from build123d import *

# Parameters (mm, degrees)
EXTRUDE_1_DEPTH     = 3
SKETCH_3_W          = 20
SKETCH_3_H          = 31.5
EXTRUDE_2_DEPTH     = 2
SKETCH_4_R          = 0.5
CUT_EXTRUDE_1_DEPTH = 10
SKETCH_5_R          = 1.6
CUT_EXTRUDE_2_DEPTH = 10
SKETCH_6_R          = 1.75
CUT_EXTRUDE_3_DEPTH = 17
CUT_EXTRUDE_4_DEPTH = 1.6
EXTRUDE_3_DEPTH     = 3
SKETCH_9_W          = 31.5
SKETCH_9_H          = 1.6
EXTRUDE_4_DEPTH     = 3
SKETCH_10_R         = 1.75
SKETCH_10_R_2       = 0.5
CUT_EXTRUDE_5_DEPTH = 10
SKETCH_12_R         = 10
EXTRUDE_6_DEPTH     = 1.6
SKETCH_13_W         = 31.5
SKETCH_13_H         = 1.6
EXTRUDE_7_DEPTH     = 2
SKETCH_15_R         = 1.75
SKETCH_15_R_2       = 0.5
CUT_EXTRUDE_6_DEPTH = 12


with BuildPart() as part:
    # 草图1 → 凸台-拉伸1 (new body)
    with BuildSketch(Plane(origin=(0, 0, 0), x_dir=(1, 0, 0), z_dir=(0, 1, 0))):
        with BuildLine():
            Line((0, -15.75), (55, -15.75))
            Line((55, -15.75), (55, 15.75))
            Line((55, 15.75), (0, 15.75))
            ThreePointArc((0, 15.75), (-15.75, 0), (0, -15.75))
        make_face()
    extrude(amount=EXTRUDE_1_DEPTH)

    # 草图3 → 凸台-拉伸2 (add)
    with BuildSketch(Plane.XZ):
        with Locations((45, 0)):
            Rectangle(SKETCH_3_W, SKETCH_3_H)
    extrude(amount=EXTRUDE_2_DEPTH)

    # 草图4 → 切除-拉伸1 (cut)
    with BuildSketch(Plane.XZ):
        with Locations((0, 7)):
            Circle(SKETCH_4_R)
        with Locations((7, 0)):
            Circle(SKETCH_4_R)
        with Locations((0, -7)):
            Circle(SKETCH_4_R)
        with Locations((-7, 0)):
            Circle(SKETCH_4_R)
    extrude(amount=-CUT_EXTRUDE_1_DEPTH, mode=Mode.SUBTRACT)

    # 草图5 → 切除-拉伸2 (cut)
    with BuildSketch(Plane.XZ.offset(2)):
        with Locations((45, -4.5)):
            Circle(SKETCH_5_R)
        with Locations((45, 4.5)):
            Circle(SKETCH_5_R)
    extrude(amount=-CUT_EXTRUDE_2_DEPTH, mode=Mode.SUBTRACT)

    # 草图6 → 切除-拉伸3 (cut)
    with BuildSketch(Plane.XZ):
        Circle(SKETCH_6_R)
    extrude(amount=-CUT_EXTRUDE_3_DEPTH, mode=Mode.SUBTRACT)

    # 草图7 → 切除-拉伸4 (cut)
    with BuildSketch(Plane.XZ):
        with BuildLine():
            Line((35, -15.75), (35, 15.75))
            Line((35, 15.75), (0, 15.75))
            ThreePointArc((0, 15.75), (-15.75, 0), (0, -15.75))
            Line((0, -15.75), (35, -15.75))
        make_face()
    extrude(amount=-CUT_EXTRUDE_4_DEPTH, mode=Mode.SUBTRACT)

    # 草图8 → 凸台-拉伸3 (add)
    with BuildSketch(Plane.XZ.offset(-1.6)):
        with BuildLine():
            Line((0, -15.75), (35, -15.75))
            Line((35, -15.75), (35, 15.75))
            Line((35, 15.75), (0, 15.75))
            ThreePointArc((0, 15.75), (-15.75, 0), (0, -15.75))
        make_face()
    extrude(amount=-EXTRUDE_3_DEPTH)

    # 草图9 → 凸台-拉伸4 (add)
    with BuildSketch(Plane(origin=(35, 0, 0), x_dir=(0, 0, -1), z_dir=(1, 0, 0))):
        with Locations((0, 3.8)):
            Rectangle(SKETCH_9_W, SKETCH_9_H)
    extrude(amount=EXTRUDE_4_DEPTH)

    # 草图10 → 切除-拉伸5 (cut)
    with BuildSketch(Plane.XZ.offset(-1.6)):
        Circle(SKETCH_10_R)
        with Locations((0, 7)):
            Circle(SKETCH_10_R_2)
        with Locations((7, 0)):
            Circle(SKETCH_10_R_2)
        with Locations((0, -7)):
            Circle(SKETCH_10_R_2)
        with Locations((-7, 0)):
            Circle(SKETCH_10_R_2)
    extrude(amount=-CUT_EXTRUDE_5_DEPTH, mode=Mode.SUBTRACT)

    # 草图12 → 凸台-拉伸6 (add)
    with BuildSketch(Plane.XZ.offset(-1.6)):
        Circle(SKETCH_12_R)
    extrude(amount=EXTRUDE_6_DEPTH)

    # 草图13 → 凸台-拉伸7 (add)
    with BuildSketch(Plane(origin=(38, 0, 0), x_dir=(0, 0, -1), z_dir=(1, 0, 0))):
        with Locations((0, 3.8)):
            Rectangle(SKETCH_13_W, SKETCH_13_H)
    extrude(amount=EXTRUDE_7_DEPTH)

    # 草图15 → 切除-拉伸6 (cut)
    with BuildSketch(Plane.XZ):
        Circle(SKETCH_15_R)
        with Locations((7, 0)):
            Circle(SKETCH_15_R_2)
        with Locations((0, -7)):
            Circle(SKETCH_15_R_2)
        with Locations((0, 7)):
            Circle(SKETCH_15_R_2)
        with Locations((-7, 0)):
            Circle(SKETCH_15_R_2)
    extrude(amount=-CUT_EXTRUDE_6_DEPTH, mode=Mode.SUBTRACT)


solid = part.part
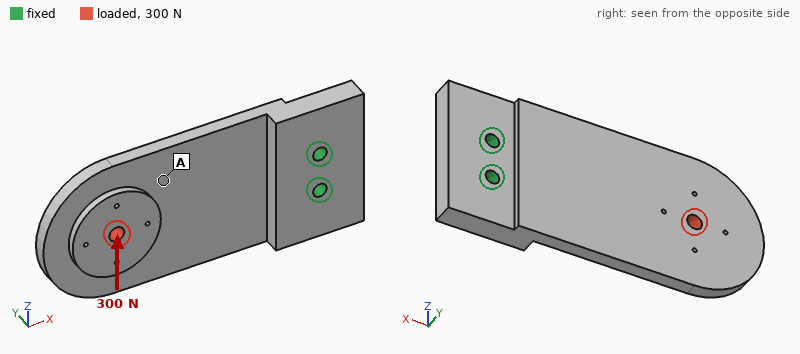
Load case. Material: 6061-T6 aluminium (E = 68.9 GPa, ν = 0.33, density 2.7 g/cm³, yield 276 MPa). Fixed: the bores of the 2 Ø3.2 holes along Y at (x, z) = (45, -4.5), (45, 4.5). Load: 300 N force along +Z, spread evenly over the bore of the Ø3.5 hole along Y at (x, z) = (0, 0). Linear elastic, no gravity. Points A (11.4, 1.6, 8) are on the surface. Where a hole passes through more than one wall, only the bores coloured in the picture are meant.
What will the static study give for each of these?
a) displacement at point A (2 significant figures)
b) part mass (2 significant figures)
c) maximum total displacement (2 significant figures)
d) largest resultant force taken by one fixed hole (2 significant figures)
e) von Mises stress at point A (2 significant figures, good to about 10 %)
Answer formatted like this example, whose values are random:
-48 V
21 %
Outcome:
32 µm
22 g
56 µm
1.2 kN
11 MPa
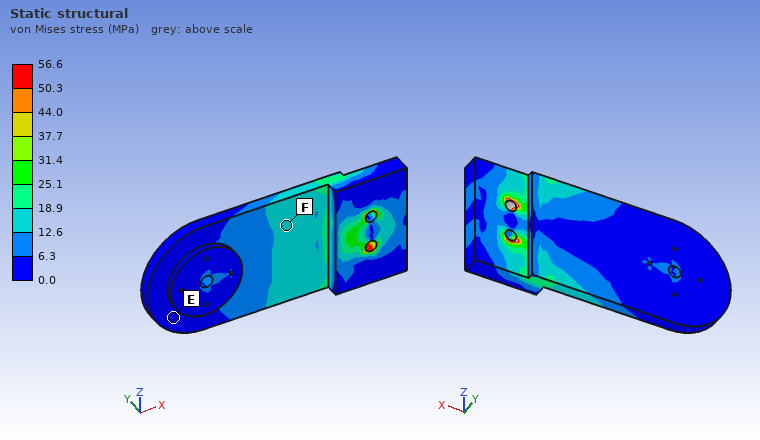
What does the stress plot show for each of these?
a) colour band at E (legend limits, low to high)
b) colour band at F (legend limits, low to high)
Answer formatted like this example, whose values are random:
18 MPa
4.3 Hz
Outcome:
0.0 to 6.3 MPa
12.6 to 18.9 MPa
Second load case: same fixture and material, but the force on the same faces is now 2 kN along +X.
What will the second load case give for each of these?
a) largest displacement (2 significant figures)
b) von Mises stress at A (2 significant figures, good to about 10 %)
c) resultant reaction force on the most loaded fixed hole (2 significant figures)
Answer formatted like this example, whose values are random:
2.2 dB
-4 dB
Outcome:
0.27 mm
51 MPa
1.0 kN
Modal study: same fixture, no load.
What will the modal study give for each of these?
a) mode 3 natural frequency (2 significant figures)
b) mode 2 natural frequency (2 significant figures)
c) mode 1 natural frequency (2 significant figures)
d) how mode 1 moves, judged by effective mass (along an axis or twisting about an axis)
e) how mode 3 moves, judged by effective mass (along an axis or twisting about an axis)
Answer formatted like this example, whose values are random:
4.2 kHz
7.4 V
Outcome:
4700 Hz
3500 Hz
890 Hz
along Y
along Z
